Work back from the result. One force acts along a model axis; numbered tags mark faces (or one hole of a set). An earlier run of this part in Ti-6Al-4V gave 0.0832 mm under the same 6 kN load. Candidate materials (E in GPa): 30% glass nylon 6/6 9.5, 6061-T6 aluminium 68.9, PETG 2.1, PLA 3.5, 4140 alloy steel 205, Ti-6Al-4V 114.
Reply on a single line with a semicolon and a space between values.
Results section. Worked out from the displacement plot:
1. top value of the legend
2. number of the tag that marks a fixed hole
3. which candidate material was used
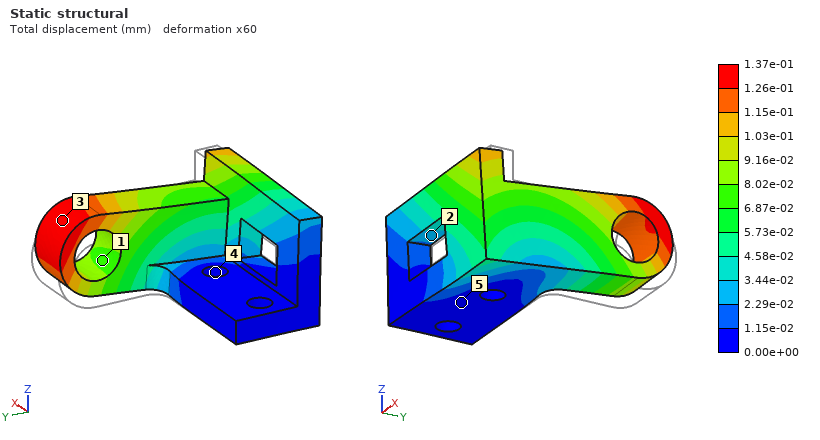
1.37e-01 mm; 4; 6061-T6 aluminium
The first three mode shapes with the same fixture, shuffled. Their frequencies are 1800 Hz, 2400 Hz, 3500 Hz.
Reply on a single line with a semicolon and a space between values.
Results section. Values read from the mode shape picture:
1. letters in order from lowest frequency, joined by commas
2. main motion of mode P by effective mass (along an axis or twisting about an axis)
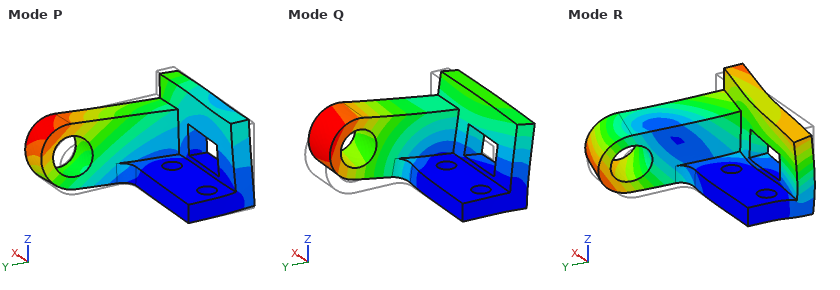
Q, P, R; along X
